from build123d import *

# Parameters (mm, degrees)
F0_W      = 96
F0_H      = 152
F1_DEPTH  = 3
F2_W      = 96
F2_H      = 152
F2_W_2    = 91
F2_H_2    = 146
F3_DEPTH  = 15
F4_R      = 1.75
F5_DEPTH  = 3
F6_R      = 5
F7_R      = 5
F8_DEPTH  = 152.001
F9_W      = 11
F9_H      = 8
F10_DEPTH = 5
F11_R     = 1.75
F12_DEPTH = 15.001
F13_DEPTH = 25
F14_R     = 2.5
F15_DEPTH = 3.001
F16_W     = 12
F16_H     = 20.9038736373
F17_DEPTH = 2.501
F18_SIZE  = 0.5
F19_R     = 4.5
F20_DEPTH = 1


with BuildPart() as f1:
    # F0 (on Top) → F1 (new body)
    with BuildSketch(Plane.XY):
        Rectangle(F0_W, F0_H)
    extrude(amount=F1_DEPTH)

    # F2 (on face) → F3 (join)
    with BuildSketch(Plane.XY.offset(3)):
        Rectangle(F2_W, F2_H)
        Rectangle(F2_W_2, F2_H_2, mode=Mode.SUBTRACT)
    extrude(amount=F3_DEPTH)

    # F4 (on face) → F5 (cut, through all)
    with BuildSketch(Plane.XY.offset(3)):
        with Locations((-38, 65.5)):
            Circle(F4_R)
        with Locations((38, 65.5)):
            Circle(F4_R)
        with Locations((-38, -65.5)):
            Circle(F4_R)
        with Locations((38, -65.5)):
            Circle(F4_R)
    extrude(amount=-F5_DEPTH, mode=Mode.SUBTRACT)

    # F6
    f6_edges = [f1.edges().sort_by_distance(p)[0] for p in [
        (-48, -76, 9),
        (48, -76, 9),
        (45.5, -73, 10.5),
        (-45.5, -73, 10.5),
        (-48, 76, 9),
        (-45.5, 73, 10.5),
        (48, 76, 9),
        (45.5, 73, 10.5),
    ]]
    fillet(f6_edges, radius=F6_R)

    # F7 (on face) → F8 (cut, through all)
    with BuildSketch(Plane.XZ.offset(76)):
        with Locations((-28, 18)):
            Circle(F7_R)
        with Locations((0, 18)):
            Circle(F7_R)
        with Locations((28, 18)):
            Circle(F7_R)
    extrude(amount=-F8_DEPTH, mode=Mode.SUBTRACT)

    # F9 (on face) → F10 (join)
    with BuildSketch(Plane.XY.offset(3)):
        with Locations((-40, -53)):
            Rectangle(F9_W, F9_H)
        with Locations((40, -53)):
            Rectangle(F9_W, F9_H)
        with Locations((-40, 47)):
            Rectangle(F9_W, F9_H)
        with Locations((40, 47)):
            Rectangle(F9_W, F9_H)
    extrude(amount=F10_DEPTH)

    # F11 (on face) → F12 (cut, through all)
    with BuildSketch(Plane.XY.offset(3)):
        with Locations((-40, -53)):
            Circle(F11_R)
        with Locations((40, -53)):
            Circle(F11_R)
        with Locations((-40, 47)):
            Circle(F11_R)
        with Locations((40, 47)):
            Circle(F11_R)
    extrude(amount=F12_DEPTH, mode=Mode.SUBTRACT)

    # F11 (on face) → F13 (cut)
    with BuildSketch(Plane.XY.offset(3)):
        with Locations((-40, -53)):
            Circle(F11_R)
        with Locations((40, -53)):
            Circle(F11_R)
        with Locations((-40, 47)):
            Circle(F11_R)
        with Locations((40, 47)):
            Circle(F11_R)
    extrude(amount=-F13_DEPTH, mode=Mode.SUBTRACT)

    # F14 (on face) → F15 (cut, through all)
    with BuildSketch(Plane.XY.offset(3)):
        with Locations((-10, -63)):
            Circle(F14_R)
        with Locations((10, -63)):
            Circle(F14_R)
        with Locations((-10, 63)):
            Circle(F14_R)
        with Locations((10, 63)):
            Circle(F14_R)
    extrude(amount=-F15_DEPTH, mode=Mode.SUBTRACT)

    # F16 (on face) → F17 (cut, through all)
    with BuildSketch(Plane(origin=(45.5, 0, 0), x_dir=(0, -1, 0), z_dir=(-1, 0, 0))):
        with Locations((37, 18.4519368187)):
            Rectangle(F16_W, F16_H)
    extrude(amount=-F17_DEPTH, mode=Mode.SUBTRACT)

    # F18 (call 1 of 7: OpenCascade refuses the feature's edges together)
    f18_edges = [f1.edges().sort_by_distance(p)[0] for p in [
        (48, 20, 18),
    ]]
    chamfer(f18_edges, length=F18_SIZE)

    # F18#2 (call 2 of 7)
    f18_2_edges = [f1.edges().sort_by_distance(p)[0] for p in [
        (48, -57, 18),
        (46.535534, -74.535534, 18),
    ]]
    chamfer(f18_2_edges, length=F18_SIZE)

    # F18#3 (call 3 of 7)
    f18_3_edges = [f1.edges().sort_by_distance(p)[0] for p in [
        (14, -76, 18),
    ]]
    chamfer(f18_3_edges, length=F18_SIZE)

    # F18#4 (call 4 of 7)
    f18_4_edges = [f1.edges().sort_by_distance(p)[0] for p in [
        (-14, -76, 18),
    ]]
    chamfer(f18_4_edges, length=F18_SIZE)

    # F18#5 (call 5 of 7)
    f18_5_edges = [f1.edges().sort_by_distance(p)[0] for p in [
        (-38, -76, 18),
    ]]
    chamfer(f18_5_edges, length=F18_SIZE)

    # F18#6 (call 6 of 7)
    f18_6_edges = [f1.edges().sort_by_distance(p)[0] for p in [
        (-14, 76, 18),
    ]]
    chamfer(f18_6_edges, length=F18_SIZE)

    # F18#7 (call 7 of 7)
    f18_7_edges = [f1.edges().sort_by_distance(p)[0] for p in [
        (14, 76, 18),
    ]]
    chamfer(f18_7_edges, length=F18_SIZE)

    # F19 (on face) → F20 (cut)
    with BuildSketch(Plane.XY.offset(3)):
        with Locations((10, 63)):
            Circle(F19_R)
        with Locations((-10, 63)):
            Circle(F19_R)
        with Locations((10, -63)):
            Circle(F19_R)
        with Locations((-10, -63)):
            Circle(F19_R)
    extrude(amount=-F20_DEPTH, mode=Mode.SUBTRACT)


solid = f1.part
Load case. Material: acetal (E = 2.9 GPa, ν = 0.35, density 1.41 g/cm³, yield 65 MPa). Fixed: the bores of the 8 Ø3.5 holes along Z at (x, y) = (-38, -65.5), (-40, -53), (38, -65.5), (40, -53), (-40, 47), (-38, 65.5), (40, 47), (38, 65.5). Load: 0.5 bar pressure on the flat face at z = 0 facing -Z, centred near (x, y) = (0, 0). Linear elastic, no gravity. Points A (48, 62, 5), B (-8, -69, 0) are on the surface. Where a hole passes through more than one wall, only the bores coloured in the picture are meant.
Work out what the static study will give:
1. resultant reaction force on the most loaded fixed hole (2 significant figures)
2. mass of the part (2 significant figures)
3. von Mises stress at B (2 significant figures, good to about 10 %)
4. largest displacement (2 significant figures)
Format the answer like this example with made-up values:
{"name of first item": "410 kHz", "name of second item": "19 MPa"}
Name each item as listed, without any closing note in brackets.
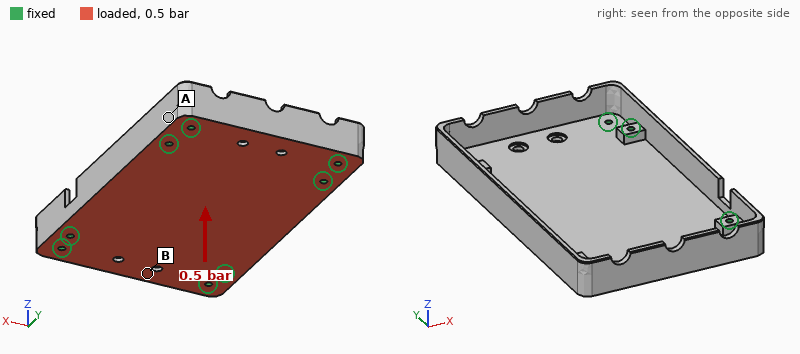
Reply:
{"resultant reaction force on the most loaded fixed hole": "190 N", "mass of the part": "89 g", "von Mises stress at B": "4.3 MPa", "largest displacement": "2.0 mm"}
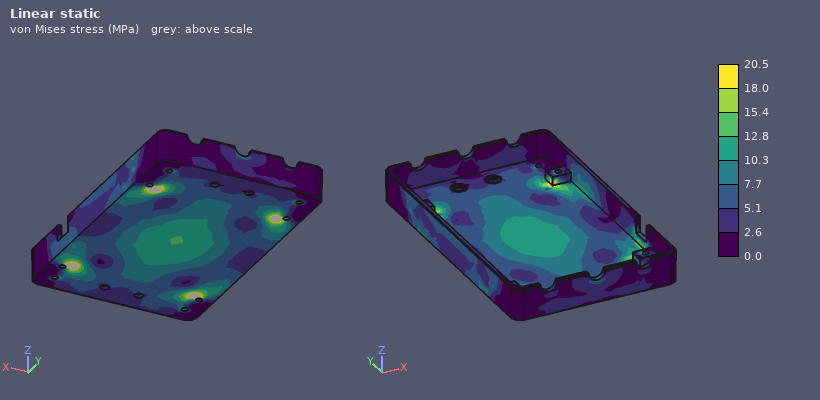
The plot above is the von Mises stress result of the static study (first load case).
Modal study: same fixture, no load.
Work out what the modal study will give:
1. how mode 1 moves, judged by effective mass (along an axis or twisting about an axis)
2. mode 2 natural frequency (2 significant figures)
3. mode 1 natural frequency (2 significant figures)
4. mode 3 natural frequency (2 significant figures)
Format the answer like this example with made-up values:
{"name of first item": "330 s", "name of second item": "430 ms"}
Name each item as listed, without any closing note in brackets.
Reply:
{"how mode 1 moves, judged by effective mass": "along Z", "mode 2 natural frequency": "910 Hz", "mode 1 natural frequency": "480 Hz", "mode 3 natural frequency": "1100 Hz"}
